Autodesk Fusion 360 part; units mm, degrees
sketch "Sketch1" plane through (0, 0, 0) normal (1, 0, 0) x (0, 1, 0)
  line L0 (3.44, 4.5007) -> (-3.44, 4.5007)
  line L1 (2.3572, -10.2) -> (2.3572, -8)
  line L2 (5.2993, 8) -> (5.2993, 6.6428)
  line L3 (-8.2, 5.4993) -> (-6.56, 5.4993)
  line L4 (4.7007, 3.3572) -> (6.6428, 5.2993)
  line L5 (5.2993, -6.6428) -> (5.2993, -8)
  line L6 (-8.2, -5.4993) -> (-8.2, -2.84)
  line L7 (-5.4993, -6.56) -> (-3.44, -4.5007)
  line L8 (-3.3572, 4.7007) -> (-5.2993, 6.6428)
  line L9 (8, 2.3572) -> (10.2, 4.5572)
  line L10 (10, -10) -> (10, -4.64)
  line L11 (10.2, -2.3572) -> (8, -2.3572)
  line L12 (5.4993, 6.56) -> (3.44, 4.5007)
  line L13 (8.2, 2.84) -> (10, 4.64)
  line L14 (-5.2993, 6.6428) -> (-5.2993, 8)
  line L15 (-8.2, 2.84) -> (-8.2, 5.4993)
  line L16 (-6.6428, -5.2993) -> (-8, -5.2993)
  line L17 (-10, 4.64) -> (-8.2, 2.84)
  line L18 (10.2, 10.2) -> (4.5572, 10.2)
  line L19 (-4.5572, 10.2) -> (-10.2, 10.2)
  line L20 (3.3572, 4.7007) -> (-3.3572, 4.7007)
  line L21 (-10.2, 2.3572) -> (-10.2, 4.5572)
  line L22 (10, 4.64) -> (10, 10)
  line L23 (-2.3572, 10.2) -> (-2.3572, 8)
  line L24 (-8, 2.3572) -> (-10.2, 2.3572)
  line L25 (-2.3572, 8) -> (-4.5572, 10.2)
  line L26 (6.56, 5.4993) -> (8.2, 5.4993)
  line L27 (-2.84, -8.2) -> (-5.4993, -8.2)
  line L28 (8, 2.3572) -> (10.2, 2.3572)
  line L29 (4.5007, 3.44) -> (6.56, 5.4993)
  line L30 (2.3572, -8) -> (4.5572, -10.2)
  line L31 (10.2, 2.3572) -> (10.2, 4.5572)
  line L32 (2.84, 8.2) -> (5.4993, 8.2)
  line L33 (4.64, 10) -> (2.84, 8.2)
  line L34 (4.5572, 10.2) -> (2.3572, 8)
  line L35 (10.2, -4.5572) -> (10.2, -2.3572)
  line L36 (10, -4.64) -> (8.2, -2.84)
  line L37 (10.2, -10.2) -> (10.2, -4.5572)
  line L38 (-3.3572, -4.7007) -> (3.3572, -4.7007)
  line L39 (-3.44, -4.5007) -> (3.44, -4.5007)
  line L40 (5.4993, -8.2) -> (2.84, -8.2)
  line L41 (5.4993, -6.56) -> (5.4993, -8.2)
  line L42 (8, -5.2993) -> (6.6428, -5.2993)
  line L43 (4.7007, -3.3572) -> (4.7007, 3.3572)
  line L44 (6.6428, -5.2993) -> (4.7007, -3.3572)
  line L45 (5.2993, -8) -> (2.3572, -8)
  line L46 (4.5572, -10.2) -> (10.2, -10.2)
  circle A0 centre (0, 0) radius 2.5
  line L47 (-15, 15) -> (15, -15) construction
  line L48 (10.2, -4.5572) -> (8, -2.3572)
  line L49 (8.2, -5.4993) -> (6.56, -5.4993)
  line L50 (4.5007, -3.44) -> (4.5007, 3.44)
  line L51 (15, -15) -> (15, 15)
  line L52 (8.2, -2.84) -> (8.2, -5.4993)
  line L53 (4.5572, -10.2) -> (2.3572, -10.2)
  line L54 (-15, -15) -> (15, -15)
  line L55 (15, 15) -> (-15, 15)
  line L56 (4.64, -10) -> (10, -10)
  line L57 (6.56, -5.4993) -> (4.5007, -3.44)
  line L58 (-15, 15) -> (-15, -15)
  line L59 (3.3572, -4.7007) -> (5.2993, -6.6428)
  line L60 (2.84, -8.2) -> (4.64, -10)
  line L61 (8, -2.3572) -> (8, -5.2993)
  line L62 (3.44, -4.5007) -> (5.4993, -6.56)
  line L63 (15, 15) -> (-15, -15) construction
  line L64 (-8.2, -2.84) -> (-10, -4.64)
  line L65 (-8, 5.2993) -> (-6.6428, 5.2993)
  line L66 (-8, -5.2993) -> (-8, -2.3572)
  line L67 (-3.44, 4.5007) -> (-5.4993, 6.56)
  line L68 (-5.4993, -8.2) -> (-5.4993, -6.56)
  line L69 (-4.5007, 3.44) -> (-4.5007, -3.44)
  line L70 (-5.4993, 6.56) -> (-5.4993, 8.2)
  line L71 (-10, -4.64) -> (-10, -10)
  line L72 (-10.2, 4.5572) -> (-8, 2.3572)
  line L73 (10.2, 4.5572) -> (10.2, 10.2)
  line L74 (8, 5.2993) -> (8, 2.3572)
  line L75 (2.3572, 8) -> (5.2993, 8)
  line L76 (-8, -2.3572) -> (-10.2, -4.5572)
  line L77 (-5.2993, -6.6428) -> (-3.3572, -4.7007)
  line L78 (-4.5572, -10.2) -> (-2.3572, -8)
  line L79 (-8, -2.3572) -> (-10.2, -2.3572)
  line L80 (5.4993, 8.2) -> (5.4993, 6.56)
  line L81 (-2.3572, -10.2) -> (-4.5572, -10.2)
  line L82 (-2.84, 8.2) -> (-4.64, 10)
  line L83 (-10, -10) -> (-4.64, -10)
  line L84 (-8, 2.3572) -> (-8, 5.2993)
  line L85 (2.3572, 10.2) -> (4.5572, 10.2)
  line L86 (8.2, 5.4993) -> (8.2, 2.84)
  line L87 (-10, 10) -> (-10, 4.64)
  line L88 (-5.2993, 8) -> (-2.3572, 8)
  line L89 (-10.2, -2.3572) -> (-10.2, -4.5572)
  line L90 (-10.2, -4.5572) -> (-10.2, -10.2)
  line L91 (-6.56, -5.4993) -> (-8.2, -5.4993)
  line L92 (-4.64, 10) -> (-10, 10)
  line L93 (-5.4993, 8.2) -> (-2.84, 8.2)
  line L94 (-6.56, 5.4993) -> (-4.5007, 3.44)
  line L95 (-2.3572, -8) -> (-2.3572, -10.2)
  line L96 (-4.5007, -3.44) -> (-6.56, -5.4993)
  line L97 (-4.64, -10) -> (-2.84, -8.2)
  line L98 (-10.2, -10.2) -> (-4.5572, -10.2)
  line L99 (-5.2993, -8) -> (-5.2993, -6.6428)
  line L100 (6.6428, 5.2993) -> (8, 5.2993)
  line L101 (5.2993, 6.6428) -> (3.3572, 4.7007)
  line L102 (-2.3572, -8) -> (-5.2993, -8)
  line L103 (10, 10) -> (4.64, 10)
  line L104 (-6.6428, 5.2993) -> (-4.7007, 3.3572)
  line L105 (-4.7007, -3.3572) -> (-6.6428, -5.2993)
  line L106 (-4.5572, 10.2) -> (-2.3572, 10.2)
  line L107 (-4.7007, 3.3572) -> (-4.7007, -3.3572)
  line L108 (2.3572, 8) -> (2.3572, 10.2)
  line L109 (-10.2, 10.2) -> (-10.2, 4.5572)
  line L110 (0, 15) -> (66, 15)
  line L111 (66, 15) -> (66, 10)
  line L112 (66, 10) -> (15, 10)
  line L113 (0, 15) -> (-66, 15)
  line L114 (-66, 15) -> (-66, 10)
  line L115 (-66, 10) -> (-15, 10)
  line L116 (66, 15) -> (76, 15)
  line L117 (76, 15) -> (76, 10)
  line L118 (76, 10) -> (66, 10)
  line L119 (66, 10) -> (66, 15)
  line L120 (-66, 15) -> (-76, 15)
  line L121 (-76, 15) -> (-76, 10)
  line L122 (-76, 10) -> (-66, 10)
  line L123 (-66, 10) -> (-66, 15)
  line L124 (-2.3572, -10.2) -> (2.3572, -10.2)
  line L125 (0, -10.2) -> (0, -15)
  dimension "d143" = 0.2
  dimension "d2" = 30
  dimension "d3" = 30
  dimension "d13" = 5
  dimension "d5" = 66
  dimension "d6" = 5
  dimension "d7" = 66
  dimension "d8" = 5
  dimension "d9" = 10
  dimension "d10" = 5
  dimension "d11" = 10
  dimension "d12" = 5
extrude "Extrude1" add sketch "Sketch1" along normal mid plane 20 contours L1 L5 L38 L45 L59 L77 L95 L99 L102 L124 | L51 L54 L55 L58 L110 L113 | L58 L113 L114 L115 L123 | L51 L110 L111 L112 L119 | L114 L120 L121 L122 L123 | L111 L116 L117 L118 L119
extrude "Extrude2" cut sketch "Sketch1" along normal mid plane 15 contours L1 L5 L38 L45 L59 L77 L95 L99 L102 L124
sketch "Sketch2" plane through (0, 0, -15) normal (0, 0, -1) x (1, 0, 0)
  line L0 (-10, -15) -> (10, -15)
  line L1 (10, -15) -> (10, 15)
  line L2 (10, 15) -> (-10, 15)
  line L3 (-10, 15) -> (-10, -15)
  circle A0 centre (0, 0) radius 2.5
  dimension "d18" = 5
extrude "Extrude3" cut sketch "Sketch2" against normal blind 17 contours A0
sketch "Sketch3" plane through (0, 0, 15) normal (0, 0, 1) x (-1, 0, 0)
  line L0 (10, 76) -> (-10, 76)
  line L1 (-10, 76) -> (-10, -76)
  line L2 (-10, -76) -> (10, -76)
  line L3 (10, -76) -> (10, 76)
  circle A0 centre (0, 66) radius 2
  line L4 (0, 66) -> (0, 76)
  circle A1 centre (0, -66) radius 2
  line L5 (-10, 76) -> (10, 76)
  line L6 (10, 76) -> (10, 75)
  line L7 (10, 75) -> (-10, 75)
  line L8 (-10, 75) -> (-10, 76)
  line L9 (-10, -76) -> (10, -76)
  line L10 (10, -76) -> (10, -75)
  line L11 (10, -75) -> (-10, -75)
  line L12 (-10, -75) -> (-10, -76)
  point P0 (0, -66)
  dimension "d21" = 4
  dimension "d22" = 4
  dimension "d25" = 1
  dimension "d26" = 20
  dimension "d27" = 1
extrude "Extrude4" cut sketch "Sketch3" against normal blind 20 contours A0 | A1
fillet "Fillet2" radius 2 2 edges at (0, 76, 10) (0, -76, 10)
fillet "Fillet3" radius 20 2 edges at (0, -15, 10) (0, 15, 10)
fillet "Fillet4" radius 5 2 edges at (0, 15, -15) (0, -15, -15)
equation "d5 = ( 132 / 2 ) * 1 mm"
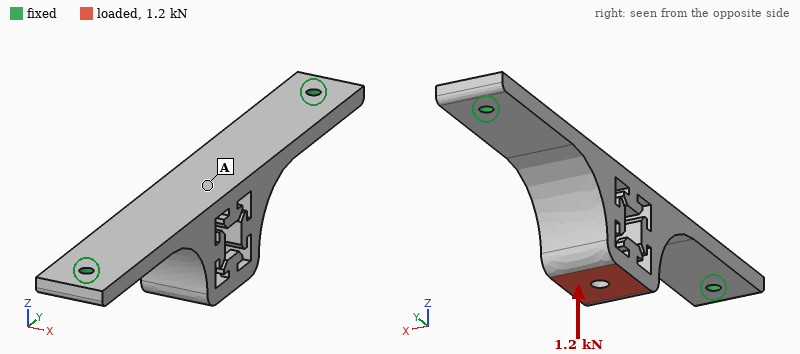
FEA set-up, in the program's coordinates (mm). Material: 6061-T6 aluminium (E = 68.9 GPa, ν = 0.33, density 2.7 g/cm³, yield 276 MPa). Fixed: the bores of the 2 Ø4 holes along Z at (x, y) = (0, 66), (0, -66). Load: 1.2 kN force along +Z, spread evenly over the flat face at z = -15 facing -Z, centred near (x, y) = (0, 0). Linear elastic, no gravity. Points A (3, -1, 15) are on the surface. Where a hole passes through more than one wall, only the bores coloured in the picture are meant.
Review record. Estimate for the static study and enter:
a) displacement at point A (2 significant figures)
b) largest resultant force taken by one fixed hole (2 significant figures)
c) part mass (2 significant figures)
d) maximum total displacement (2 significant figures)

0.28 mm
890 N
74 g
0.28 mm
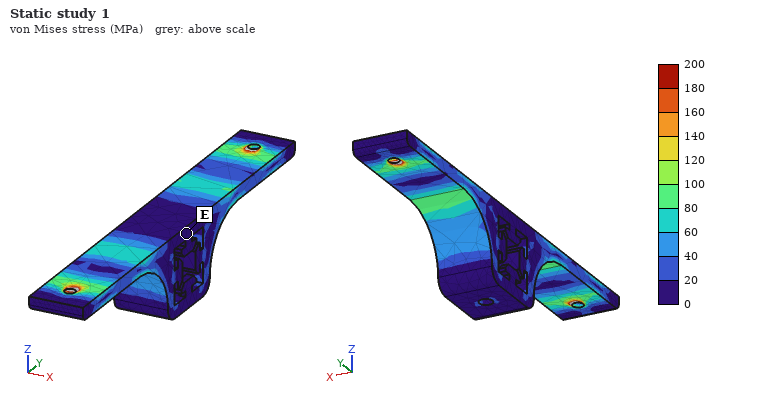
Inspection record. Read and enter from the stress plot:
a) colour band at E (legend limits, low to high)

0 to 20 MPa
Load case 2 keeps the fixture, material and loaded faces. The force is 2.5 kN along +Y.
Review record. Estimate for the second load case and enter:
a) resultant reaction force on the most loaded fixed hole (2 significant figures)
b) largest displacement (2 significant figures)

1.4 kN
0.21 mm
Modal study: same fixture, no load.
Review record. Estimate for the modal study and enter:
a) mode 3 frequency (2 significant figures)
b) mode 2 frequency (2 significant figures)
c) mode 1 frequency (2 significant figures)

3300 Hz
1400 Hz
1400 Hz
